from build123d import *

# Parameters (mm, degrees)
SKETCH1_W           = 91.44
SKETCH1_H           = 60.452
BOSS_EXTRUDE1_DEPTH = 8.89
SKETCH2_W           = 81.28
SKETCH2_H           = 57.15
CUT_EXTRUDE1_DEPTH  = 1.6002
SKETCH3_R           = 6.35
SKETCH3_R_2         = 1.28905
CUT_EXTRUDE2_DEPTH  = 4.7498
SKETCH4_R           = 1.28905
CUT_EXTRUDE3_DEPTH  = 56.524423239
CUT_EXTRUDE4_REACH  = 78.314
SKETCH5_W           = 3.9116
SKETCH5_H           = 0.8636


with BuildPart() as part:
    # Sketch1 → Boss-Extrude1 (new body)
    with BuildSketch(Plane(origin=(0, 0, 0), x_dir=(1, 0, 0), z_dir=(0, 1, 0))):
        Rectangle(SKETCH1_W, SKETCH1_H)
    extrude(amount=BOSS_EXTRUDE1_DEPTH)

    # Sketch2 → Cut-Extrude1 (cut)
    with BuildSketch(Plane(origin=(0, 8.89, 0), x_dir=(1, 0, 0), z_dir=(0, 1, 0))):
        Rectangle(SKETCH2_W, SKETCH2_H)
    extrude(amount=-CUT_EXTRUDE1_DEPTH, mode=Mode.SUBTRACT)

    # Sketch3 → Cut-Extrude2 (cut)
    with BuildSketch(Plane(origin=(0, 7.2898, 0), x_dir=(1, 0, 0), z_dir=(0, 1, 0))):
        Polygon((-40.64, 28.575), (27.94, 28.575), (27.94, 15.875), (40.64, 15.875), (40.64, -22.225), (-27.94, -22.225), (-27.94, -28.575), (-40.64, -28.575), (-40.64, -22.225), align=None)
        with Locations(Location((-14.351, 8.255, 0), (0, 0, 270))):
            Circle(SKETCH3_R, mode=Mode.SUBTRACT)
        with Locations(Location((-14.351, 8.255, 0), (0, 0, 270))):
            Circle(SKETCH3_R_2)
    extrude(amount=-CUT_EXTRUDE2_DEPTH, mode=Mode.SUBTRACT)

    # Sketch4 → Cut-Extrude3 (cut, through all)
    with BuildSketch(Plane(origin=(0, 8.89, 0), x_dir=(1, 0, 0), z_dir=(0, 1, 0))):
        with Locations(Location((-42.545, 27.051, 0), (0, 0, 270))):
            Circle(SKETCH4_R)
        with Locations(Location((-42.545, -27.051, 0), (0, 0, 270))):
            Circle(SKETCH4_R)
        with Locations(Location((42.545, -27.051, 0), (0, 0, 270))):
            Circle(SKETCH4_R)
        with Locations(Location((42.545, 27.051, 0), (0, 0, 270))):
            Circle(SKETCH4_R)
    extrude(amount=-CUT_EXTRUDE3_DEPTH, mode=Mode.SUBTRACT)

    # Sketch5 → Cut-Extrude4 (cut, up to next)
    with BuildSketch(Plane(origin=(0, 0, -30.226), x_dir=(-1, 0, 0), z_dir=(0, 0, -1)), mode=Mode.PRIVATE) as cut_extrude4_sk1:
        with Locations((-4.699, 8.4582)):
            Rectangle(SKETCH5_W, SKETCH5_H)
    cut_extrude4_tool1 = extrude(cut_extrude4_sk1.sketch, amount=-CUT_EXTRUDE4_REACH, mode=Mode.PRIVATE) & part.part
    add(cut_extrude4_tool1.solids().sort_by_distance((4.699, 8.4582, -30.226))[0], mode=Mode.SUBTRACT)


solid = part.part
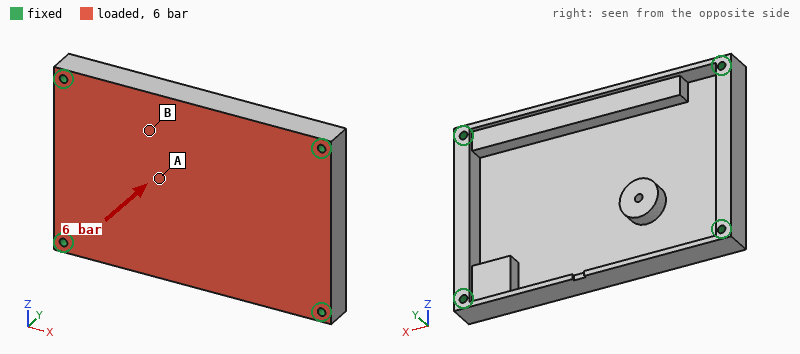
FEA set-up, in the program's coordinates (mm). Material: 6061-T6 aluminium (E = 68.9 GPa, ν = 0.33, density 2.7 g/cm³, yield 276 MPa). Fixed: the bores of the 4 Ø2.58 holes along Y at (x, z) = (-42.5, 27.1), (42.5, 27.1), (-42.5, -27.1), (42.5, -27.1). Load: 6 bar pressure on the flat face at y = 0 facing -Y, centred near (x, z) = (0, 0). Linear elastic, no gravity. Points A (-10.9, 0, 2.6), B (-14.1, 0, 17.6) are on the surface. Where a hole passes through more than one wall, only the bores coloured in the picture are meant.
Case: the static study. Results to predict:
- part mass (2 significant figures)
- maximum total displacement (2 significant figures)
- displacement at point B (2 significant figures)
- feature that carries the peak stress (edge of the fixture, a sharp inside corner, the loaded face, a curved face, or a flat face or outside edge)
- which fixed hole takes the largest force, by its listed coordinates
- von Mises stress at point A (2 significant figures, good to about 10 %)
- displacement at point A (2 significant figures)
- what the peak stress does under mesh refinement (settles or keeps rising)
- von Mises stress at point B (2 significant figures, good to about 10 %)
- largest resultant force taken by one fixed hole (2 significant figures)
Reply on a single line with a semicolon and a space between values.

62 g; 0.31 mm; 0.18 mm; edge of the fixture; (42.5, -27.1); 82 MPa; 0.28 mm; keeps rising; 40 MPa; 1.2 kN
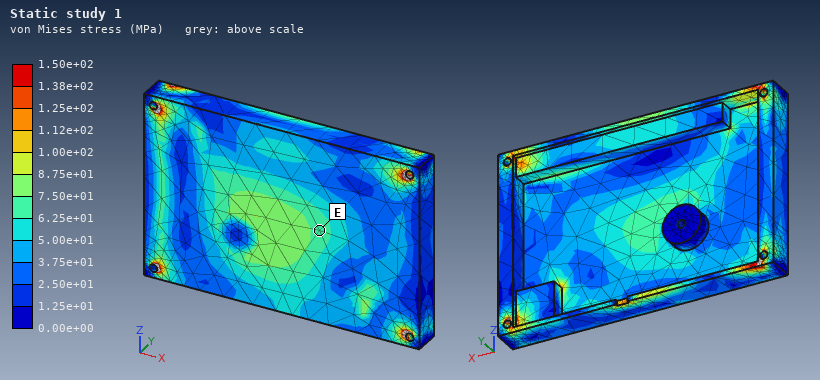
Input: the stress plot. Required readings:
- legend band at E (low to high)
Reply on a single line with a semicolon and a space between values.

6.25e+01 to 7.50e+01 MPa
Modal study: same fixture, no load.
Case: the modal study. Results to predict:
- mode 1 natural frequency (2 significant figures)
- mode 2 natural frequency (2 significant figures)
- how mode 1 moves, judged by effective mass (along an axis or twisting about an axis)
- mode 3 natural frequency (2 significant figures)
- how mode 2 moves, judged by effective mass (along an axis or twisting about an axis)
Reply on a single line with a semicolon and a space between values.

3100 Hz; 4900 Hz; along Y; 6500 Hz; twisting about X
